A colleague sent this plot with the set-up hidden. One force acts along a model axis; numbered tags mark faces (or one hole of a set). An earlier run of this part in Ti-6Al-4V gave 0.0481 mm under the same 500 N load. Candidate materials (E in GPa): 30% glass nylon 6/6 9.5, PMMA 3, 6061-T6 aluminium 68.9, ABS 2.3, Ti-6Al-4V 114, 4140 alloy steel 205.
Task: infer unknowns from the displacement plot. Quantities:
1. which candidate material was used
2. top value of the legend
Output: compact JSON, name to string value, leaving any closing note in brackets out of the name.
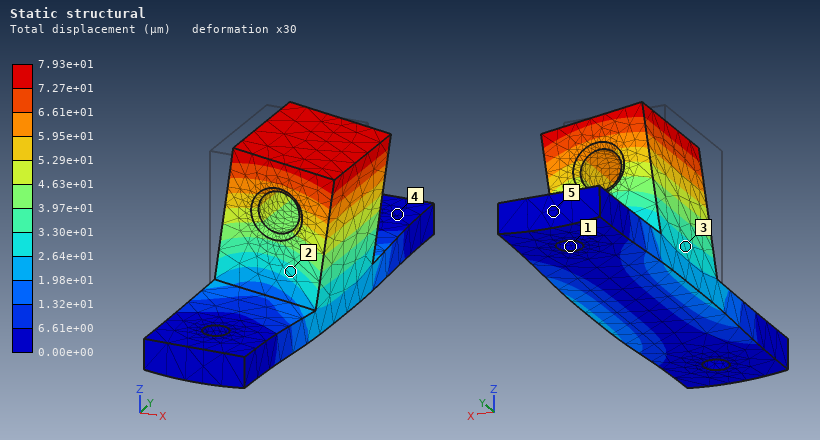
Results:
{"which candidate material was used": "6061-T6 aluminium", "top value of the legend": "7.93e+01 µm"}
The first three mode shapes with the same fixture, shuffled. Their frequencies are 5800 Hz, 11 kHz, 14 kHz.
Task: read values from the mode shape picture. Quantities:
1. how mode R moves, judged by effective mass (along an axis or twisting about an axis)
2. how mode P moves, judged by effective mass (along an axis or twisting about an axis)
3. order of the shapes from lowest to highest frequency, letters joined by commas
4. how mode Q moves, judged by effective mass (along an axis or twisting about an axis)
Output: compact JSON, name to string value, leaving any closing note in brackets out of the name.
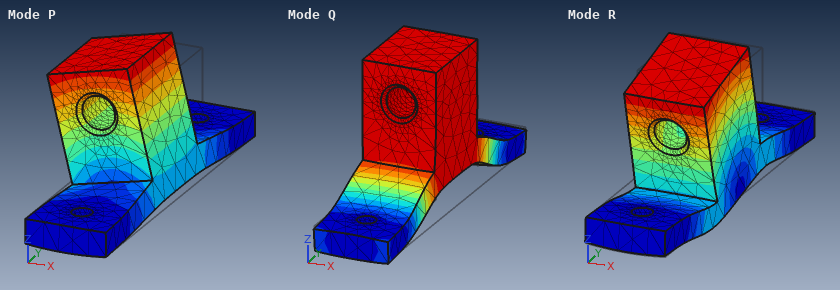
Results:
{"how mode R moves, judged by effective mass": "along Y", "how mode P moves, judged by effective mass": "along X", "order of the shapes from lowest to highest frequency, letters joined by commas": "P, Q, R", "how mode Q moves, judged by effective mass": "along Z"}
